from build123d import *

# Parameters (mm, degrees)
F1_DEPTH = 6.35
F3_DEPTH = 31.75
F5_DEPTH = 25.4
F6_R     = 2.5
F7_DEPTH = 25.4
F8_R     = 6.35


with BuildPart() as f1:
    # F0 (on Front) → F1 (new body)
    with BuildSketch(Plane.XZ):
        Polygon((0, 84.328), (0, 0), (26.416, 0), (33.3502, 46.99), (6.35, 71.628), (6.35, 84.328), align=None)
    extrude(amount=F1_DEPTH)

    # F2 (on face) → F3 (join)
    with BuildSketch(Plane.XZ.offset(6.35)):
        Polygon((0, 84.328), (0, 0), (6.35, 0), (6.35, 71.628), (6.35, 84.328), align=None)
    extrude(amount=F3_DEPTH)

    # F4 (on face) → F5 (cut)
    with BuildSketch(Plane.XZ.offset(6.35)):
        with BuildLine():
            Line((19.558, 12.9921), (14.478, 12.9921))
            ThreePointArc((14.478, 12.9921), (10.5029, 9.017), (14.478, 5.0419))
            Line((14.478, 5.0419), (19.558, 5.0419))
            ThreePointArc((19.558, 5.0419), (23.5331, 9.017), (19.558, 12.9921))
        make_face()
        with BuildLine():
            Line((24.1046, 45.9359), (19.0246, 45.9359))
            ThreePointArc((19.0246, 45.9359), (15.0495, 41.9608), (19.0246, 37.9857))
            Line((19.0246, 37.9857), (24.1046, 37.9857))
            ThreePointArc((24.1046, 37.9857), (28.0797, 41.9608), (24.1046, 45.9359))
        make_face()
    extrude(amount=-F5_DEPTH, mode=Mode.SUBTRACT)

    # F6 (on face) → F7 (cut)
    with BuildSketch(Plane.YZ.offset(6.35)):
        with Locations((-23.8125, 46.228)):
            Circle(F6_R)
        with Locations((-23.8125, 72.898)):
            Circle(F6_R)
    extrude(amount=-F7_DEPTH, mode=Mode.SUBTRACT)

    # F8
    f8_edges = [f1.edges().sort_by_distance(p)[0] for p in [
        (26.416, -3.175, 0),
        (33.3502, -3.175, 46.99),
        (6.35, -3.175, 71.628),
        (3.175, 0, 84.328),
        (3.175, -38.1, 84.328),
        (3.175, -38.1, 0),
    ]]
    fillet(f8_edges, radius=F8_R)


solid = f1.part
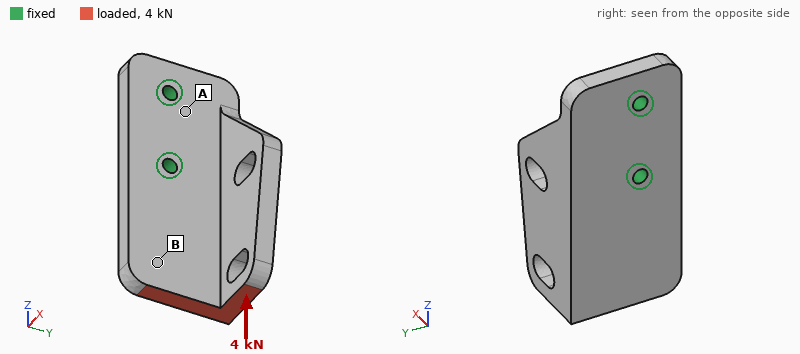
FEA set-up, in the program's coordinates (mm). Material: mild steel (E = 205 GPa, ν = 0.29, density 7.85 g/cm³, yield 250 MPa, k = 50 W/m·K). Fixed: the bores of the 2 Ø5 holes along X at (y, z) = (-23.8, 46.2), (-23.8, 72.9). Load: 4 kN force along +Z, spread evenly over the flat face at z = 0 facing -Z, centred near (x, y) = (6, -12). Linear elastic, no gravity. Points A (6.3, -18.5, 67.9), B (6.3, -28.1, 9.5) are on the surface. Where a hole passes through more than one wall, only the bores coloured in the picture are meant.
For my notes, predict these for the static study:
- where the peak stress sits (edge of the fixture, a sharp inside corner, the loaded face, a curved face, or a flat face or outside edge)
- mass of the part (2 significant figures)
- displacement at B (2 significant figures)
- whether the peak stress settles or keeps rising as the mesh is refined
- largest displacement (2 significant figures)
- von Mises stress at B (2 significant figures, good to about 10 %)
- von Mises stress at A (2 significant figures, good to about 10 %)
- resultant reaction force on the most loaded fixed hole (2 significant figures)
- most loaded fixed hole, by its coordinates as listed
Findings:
edge of the fixture
220 g
9.8 µm
keeps rising
25 µm
12 MPa
32 MPa
3.1 kN
(-23.8, 46.2)
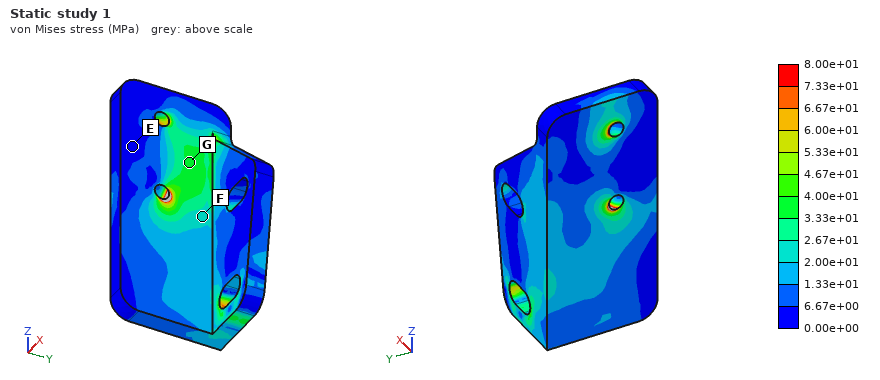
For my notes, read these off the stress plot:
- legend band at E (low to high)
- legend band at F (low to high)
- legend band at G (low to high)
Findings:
0.00e+00 to 6.67e+00 MPa
2.00e+01 to 2.67e+01 MPa
3.33e+01 to 4.00e+01 MPa
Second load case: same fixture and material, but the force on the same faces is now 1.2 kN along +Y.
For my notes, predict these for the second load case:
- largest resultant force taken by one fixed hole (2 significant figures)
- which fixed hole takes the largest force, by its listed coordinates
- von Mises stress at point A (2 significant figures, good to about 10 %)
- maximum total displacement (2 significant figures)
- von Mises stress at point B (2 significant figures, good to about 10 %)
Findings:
2.9 kN
(-23.8, 46.2)
20 MPa
40 µm
14 MPa
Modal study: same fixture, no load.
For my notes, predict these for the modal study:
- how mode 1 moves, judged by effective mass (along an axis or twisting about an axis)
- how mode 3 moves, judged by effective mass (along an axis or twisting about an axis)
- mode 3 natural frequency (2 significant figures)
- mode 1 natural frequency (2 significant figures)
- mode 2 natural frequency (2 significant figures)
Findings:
along X
along Y
5900 Hz
2200 Hz
3400 Hz
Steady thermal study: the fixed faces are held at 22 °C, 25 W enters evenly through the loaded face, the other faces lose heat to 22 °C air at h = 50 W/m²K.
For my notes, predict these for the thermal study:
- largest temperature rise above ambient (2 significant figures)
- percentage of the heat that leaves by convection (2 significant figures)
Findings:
69 K
45 %
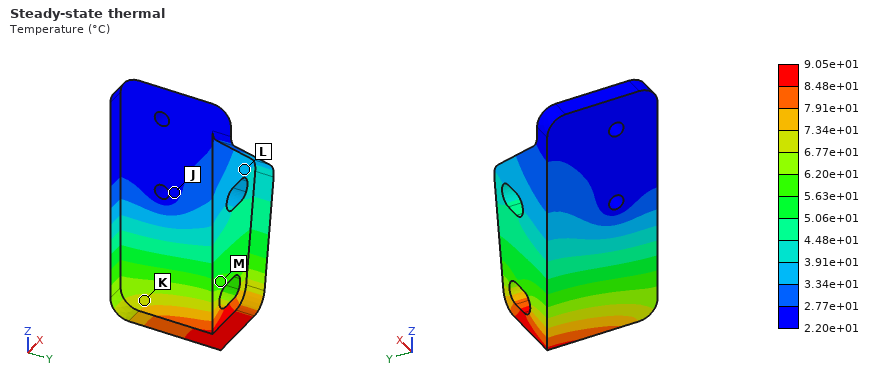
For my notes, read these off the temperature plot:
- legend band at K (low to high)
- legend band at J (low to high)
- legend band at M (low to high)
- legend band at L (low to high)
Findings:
6.77e+01 to 7.34e+01 °C
2.20e+01 to 2.77e+01 °C
5.63e+01 to 6.20e+01 °C
3.34e+01 to 3.91e+01 °C
